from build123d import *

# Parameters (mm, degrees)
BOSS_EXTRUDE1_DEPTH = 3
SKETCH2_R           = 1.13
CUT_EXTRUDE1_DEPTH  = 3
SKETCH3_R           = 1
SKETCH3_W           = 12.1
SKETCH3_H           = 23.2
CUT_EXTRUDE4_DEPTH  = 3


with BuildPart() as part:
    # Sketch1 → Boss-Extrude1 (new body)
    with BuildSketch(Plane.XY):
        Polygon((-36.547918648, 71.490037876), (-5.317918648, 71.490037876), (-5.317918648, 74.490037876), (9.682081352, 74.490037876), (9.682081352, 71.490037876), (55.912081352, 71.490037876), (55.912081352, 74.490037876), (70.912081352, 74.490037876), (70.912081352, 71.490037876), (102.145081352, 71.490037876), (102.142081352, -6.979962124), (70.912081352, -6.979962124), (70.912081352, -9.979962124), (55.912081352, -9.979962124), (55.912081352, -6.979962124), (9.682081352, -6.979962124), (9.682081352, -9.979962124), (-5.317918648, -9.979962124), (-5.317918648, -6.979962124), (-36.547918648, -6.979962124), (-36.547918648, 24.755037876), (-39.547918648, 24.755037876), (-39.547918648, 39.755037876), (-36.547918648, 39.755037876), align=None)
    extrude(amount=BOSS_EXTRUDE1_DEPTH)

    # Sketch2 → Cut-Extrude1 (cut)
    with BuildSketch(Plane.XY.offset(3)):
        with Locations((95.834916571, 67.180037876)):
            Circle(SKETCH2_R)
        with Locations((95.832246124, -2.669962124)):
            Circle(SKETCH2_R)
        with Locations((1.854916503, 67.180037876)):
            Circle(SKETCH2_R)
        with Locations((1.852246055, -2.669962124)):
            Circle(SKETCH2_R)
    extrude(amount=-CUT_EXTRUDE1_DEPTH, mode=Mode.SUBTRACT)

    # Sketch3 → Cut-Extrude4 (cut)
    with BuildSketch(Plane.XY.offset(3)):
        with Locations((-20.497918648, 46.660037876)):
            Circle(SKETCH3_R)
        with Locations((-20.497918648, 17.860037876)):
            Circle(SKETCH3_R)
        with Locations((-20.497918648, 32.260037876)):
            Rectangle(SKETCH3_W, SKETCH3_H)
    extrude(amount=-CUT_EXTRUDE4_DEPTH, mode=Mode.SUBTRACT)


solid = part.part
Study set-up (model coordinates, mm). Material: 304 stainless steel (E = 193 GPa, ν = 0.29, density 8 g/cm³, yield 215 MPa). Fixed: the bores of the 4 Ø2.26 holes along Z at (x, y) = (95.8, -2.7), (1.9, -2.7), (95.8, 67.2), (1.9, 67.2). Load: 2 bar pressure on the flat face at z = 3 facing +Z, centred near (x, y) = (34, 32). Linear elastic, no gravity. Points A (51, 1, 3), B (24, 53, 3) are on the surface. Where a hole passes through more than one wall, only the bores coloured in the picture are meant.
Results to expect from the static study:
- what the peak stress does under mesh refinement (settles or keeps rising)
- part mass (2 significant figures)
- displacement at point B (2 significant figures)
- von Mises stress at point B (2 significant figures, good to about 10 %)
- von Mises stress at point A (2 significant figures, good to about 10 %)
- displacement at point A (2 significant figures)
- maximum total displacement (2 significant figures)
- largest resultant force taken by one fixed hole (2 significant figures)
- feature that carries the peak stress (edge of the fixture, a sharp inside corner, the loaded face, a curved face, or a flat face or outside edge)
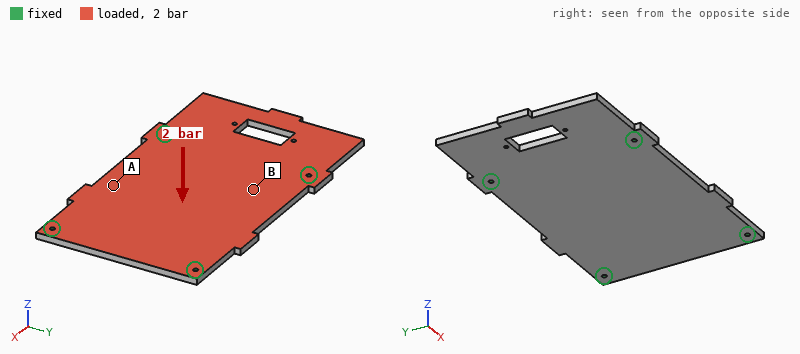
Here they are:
keeps rising
260 g
0.098 mm
27 MPa
63 MPa
0.14 mm
0.20 mm
680 N
edge of the fixture
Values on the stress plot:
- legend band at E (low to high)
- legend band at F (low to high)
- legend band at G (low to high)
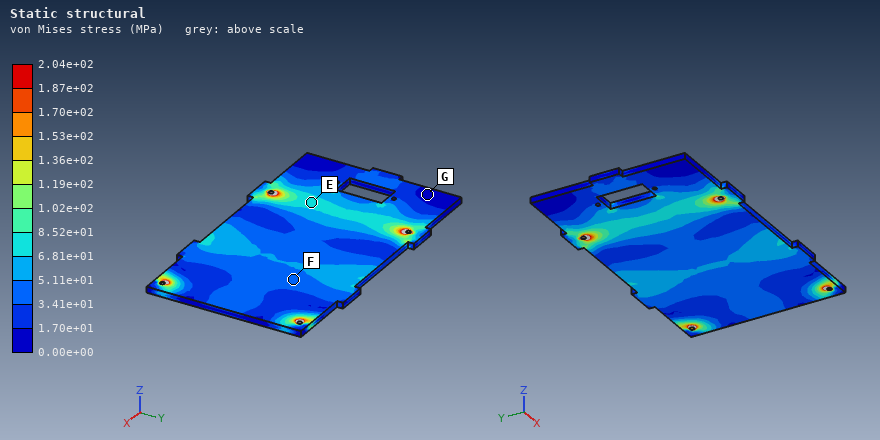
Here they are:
6.81e+01 to 8.52e+01 MPa
3.41e+01 to 5.11e+01 MPa
0.00e+00 to 1.70e+01 MPa
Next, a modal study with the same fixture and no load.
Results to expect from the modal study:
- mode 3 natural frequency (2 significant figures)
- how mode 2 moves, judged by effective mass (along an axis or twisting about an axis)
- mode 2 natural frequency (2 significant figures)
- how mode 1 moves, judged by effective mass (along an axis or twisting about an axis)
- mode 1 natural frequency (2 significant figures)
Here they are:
2000 Hz
along Z
1300 Hz
twisting about Y
1100 Hz
